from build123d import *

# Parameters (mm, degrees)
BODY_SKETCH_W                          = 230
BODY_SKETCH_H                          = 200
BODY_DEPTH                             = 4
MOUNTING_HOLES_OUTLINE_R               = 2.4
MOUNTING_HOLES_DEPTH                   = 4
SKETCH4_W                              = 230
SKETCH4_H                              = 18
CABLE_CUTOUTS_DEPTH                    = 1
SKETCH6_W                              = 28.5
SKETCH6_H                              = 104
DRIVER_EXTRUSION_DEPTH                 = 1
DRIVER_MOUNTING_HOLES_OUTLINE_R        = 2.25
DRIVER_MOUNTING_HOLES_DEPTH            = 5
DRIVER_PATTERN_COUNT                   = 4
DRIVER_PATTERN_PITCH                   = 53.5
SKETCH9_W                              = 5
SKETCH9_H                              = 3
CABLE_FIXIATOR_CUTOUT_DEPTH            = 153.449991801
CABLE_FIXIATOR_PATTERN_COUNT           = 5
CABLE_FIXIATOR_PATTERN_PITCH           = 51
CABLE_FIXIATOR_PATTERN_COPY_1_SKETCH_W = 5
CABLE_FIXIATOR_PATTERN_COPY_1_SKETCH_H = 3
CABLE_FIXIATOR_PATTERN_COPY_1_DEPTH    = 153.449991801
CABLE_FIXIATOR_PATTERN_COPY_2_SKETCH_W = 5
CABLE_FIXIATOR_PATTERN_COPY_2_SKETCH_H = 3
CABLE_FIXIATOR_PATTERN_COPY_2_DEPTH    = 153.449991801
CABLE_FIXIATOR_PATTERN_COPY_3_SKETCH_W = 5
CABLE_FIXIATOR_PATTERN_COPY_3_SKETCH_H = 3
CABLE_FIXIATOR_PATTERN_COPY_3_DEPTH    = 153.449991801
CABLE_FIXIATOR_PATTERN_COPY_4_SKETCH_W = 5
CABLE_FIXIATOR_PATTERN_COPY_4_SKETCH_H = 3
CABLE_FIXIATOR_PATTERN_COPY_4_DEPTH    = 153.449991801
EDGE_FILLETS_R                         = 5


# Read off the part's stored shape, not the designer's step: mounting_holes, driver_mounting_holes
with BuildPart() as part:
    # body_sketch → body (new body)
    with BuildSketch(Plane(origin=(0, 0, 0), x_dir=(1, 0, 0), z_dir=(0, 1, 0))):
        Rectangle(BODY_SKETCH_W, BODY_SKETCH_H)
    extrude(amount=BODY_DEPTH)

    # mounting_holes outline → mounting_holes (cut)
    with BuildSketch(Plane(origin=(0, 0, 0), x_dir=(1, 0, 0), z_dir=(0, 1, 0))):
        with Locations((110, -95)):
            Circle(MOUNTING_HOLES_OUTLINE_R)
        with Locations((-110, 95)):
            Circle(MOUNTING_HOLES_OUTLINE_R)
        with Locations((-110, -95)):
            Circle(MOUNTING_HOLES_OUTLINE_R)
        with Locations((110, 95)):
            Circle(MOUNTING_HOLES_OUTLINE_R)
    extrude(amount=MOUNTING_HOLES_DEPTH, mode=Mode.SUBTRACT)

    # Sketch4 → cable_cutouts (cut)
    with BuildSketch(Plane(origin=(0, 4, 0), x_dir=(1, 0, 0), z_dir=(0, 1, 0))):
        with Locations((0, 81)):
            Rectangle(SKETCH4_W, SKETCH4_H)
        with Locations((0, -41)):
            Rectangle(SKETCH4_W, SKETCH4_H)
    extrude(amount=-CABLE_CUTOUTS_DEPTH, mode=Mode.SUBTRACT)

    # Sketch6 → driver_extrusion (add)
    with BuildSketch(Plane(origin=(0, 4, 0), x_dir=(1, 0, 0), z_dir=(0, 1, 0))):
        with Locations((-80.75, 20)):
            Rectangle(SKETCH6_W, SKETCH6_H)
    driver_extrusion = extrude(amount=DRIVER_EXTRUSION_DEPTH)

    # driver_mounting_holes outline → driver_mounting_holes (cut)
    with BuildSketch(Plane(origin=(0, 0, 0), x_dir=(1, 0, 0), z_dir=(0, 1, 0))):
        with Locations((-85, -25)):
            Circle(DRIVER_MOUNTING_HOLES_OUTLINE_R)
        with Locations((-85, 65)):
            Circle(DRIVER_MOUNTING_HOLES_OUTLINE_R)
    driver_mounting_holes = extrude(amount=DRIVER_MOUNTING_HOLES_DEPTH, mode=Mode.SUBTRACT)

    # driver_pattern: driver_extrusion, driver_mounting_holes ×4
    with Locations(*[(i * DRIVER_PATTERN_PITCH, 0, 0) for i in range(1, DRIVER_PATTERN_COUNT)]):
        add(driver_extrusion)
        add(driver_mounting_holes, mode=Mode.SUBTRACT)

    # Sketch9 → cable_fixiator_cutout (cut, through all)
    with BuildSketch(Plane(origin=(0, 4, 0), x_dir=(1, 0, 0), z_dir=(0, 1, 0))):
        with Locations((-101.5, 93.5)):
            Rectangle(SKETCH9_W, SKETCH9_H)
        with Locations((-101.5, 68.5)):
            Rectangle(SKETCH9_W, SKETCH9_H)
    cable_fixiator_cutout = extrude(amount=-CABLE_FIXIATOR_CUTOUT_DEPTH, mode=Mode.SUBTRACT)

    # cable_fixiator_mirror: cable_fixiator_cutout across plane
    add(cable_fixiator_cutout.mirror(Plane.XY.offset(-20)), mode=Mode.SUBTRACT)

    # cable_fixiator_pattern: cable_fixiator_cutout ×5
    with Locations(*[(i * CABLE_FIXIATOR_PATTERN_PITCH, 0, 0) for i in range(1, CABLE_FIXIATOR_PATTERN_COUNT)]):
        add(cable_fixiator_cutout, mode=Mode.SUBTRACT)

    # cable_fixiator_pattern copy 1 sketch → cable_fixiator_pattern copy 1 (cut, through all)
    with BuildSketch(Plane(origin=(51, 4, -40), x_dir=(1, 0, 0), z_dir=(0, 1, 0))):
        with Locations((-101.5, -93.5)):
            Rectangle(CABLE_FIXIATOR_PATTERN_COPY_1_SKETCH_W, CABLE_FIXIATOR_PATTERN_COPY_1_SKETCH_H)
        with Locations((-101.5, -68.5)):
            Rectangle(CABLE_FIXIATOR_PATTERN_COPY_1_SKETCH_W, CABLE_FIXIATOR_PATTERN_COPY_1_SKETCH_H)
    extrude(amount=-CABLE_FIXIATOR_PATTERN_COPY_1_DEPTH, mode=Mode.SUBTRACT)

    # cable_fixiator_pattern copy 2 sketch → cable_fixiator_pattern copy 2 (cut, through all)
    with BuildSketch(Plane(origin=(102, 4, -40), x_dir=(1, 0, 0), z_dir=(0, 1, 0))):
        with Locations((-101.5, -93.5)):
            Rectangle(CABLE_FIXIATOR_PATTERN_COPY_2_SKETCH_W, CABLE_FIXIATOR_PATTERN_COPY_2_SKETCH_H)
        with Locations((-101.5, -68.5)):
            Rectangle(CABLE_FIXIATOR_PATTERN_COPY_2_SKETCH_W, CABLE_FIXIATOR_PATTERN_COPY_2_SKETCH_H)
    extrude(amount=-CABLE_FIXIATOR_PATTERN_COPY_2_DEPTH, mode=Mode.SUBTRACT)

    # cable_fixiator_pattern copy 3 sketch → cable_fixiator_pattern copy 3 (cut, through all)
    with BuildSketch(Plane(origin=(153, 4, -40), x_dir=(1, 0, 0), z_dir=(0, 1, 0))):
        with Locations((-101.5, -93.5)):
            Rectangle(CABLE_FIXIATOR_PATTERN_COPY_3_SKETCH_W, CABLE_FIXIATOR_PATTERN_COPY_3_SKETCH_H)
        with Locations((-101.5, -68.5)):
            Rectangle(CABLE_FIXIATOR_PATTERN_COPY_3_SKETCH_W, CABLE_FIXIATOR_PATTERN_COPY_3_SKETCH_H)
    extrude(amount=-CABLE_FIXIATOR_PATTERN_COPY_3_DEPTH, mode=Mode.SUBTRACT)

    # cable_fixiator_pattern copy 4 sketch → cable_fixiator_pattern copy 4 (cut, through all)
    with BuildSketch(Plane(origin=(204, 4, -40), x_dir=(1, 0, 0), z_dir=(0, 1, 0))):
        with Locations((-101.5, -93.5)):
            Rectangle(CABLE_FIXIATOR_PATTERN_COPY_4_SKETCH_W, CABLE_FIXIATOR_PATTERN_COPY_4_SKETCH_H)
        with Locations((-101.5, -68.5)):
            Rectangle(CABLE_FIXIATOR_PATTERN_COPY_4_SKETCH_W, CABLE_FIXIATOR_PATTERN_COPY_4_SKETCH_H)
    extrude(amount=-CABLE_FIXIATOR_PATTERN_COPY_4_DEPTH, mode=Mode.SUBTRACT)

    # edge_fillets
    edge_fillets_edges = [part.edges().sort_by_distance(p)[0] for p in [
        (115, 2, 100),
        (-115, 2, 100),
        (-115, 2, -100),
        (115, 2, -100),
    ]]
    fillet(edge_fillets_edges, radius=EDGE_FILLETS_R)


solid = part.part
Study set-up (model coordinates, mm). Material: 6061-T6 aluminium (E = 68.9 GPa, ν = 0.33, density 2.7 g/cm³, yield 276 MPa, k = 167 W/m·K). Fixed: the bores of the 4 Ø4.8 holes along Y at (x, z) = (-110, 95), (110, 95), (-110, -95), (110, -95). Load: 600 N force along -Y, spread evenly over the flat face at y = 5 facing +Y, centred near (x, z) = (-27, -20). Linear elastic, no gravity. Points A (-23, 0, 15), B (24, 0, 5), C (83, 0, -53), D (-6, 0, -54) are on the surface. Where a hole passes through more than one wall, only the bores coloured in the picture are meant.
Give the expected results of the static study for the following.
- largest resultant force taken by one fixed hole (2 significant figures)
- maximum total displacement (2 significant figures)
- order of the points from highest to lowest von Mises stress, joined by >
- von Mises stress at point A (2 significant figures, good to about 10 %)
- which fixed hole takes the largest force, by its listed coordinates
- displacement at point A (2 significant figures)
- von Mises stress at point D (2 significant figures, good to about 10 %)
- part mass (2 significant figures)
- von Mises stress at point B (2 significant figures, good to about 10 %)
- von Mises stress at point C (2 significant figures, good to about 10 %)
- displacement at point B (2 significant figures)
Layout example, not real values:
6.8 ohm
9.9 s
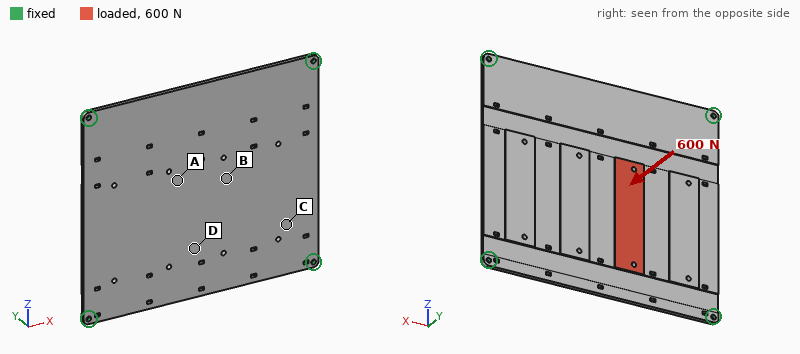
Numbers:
330 N
0.99 mm
D > A > B > C
26 MPa
(-110, -95)
0.94 mm
37 MPa
500 g
14 MPa
8.3 MPa
0.83 mm
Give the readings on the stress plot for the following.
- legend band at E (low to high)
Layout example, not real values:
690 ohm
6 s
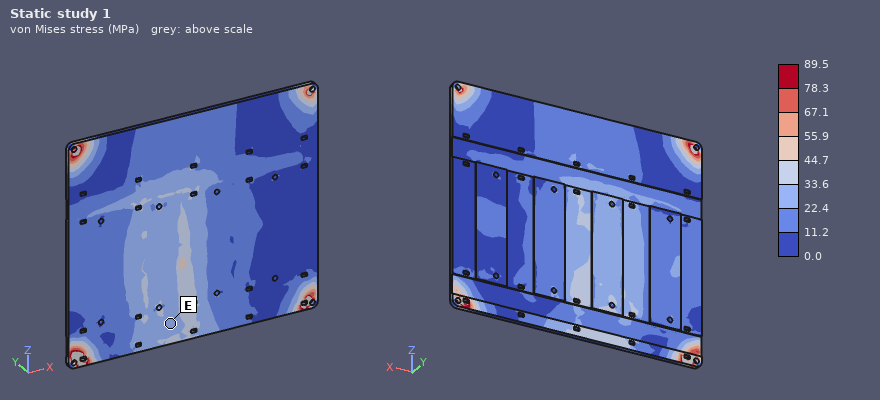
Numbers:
22.4 to 33.6 MPa
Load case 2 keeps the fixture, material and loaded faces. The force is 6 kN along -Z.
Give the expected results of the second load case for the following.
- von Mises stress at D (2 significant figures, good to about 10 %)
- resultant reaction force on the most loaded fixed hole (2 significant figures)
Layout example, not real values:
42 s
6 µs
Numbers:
9.1 MPa
2.1 kN
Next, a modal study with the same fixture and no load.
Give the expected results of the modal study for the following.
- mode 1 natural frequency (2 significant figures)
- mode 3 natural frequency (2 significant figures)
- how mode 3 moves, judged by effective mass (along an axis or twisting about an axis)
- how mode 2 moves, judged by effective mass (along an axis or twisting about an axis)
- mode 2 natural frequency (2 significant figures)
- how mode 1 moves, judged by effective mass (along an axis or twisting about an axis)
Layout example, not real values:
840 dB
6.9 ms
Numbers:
260 Hz
530 Hz
twisting about Z
twisting about X
480 Hz
along Y
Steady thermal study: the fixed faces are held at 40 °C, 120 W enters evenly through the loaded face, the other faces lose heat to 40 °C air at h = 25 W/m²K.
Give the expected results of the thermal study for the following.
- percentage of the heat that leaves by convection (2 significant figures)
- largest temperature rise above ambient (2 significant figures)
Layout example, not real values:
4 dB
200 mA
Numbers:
61 %
63 K
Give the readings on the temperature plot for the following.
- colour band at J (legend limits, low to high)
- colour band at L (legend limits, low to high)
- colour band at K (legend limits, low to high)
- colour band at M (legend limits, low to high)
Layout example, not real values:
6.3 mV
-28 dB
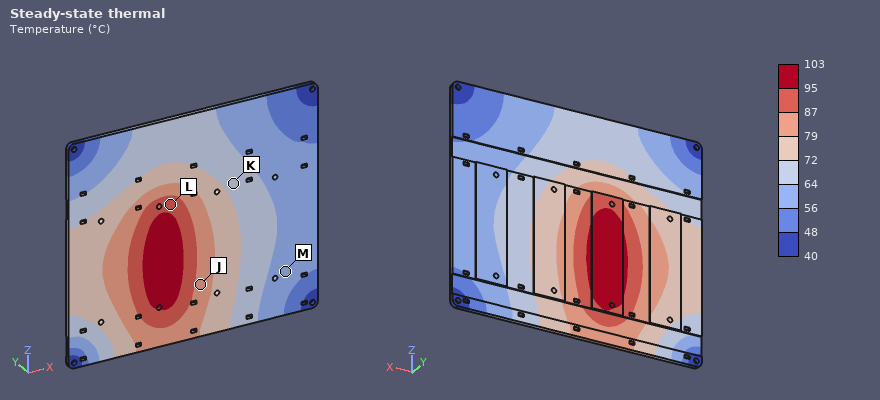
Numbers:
79 to 87 °C
87 to 95 °C
64 to 72 °C
56 to 64 °C
